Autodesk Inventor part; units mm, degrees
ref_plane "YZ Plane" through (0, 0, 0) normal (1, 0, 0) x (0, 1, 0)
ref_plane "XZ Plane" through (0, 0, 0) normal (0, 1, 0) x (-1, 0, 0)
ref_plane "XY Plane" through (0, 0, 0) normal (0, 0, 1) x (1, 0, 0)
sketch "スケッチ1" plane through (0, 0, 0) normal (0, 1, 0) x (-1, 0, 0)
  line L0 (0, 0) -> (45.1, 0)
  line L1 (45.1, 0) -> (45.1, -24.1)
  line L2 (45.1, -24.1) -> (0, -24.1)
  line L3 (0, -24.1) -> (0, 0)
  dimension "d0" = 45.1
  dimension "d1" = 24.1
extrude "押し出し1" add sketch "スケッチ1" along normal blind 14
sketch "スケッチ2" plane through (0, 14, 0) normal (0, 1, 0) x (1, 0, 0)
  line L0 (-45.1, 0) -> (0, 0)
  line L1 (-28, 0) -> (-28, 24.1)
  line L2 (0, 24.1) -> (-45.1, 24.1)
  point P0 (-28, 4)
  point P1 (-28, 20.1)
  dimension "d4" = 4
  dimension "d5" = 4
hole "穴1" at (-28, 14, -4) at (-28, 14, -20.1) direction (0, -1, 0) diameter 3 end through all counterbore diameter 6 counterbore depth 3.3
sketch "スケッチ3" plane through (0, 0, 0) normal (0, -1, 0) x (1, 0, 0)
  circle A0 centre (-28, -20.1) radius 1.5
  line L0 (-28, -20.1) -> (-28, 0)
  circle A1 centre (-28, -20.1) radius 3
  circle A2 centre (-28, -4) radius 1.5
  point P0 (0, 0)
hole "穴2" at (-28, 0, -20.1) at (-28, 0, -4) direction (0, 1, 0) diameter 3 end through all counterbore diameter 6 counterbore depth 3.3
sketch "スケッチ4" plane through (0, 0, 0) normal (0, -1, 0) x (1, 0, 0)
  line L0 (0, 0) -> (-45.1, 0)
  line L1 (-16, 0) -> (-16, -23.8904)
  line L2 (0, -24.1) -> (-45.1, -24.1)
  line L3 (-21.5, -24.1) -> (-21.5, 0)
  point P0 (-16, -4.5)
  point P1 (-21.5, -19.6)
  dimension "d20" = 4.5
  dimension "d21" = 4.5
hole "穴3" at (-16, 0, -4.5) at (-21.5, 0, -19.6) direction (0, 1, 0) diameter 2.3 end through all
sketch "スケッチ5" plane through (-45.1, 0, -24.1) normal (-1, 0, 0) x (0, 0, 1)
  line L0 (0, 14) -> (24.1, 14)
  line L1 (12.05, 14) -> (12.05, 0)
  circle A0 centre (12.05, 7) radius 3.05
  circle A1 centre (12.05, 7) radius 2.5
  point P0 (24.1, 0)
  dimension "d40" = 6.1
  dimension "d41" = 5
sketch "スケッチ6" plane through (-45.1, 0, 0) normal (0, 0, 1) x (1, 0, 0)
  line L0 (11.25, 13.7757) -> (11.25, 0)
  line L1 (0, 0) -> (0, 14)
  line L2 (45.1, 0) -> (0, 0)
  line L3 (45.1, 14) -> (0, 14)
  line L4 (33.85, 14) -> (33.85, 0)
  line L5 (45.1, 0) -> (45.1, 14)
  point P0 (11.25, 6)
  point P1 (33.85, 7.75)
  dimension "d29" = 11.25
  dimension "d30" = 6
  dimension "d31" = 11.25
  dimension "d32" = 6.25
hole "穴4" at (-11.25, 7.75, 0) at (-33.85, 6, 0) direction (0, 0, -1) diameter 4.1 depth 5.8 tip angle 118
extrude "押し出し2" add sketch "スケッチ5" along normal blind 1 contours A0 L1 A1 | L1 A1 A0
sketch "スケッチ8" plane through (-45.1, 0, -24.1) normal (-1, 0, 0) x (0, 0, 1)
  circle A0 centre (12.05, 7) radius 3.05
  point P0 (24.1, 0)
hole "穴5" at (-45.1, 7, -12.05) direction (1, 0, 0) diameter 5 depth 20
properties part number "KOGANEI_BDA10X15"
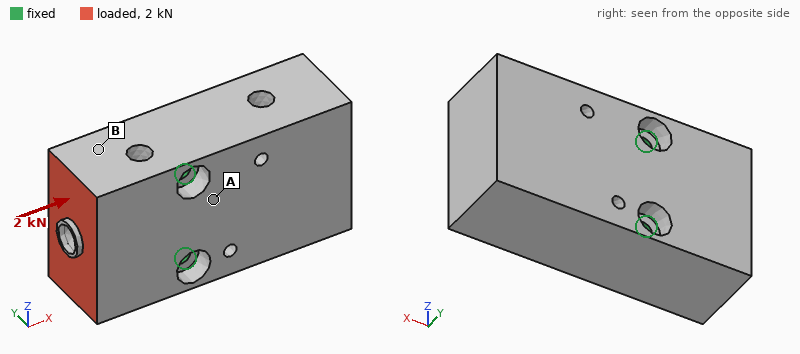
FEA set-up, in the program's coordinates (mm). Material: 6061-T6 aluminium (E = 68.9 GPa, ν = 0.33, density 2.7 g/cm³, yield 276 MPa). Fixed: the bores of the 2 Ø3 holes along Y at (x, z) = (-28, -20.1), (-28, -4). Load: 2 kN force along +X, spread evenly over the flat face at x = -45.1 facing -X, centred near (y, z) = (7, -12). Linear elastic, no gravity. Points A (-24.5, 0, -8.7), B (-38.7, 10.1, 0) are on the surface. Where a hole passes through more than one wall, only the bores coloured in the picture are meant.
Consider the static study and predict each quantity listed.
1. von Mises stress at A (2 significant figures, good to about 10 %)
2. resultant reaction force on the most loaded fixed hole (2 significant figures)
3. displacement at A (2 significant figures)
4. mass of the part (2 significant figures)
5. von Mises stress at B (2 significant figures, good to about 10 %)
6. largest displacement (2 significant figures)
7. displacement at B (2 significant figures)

3.4 MPa
1.0 kN
0.78 µm
38 g
8.7 MPa
2.8 µm
1.9 µm
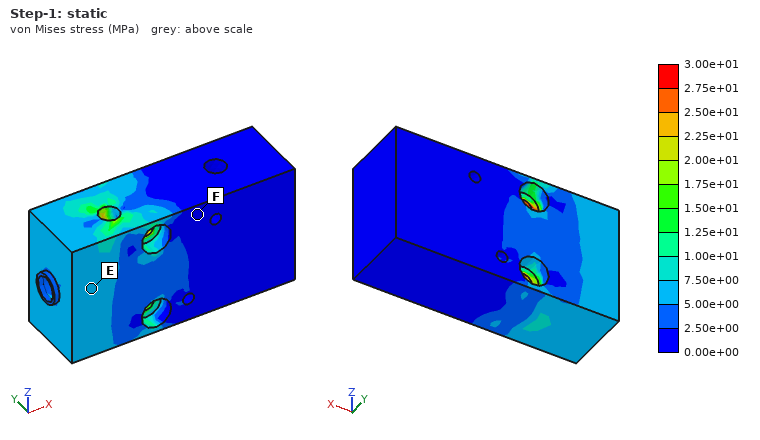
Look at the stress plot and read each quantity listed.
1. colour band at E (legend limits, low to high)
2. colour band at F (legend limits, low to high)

5.00e+00 to 7.50e+00 MPa
0.00e+00 to 2.50e+00 MPa
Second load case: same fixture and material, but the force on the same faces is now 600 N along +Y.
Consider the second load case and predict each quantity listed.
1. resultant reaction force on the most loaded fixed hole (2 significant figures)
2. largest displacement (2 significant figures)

300 N
14 µm
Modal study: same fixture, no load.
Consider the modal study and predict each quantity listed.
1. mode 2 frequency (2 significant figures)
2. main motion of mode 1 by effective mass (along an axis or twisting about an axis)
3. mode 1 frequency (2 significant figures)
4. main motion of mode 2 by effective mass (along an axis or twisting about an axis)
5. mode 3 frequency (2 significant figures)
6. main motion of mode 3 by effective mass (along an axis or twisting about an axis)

15 kHz
along Y
7000 Hz
along Z
19 kHz
along Y
